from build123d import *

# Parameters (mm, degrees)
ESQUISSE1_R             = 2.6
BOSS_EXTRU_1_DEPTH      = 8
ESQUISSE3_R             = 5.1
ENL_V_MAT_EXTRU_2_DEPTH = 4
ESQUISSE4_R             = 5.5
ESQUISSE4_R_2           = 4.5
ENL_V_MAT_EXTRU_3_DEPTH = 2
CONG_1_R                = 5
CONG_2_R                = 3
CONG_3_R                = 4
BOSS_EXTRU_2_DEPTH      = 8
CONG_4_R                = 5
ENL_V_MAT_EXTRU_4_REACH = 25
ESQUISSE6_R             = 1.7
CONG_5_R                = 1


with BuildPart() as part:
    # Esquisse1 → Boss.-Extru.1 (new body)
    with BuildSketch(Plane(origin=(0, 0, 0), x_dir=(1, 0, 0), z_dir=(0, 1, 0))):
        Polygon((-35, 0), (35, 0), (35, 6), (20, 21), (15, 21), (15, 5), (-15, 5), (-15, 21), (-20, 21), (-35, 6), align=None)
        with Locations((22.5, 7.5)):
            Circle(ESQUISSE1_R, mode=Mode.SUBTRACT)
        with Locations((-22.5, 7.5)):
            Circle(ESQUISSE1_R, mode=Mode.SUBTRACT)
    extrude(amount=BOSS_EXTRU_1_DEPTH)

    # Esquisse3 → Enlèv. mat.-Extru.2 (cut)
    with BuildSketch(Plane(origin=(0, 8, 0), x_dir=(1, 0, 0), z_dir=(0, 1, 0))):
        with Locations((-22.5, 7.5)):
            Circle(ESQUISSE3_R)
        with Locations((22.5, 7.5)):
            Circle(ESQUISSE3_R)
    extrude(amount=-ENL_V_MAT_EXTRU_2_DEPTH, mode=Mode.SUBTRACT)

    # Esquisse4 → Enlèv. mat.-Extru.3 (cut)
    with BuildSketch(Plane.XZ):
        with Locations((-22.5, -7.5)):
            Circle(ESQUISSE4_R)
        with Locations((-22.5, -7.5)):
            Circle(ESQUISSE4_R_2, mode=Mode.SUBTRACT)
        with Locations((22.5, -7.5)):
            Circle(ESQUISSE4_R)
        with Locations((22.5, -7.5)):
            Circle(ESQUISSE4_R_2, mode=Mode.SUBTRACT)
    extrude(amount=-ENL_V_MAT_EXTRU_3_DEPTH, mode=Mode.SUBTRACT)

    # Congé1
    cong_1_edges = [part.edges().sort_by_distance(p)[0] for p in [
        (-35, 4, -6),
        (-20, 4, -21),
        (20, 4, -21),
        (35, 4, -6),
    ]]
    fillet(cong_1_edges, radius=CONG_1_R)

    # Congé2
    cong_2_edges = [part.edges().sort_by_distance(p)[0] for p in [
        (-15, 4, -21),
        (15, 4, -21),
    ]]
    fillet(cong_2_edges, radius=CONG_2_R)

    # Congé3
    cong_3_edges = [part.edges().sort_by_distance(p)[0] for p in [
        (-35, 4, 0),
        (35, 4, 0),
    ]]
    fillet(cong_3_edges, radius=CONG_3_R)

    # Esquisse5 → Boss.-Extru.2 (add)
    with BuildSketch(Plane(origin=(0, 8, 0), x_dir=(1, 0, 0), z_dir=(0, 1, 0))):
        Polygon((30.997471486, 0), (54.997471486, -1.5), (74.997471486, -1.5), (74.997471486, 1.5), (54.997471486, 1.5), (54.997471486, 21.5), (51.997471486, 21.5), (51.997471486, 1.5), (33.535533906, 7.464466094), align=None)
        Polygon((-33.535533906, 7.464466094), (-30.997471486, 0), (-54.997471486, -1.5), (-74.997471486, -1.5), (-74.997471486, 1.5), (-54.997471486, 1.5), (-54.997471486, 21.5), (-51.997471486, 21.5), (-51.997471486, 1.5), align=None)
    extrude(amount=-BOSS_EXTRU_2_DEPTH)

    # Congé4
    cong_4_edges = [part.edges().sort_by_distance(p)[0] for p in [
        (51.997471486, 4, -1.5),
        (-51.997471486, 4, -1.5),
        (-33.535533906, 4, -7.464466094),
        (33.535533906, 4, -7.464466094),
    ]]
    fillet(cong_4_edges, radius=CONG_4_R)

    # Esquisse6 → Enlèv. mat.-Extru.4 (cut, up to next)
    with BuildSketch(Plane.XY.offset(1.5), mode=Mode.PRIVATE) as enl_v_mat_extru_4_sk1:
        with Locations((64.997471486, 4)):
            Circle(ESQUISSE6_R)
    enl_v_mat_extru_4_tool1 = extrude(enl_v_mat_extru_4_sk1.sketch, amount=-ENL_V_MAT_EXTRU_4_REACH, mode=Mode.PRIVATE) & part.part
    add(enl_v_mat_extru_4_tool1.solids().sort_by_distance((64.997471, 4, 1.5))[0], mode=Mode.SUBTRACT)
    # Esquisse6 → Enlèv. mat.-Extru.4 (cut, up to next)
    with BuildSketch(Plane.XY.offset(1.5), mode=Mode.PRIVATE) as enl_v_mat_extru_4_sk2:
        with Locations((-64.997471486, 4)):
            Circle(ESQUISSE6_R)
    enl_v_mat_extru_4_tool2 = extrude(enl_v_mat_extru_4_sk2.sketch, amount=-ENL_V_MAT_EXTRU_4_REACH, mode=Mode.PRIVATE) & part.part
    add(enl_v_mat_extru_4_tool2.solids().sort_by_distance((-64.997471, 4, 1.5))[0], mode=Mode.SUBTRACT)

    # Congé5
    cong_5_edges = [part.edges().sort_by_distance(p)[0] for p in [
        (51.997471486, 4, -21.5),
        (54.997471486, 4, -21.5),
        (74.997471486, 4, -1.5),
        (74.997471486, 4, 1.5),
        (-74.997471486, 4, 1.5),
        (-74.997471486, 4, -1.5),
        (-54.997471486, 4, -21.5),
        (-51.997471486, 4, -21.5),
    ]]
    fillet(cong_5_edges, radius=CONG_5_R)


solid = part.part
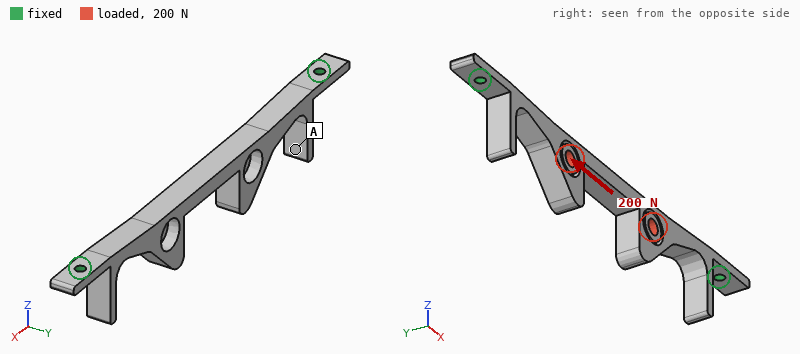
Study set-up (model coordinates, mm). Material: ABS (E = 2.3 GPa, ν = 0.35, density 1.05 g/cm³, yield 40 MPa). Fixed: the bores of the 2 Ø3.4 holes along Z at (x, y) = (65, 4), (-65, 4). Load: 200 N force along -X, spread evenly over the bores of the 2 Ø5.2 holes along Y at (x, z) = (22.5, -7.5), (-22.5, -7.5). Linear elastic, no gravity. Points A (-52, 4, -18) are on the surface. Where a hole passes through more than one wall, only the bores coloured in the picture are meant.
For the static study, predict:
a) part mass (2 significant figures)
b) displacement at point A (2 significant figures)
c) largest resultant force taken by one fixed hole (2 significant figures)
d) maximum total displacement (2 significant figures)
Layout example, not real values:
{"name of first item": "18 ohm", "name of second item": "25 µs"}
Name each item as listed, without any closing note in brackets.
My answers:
{"part mass": "9.1 g", "displacement at point A": "0.070 mm", "largest resultant force taken by one fixed hole": "100 N", "maximum total displacement": "0.14 mm"}
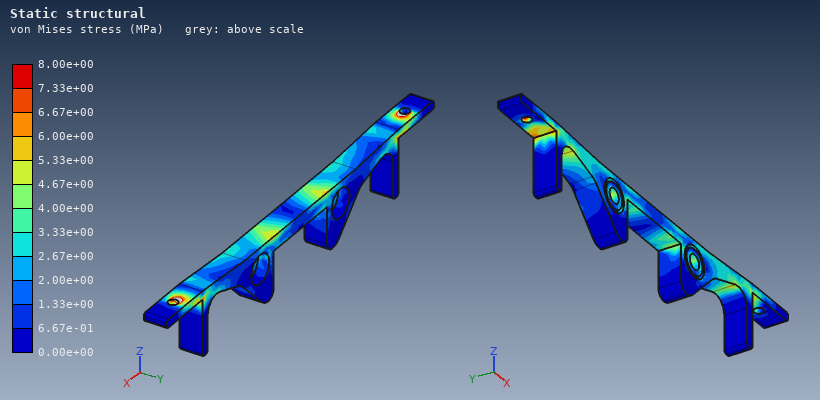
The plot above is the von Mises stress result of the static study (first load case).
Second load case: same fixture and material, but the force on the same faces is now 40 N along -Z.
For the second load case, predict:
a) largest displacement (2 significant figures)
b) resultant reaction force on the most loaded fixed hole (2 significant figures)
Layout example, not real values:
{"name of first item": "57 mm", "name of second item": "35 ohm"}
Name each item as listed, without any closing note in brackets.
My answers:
{"largest displacement": "1.8 mm", "resultant reaction force on the most loaded fixed hole": "110 N"}
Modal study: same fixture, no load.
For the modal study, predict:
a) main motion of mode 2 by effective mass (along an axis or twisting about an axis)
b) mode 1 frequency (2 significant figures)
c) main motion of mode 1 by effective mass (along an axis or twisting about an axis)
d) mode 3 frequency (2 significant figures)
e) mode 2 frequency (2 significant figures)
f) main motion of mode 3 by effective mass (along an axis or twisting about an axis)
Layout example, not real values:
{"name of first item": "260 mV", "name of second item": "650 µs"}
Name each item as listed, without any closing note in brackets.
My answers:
{"main motion of mode 2 by effective mass": "along Y", "mode 1 frequency": "340 Hz", "main motion of mode 1 by effective mass": "along Z", "mode 3 frequency": "890 Hz", "mode 2 frequency": "390 Hz", "main motion of mode 3 by effective mass": "twisting about X"}
